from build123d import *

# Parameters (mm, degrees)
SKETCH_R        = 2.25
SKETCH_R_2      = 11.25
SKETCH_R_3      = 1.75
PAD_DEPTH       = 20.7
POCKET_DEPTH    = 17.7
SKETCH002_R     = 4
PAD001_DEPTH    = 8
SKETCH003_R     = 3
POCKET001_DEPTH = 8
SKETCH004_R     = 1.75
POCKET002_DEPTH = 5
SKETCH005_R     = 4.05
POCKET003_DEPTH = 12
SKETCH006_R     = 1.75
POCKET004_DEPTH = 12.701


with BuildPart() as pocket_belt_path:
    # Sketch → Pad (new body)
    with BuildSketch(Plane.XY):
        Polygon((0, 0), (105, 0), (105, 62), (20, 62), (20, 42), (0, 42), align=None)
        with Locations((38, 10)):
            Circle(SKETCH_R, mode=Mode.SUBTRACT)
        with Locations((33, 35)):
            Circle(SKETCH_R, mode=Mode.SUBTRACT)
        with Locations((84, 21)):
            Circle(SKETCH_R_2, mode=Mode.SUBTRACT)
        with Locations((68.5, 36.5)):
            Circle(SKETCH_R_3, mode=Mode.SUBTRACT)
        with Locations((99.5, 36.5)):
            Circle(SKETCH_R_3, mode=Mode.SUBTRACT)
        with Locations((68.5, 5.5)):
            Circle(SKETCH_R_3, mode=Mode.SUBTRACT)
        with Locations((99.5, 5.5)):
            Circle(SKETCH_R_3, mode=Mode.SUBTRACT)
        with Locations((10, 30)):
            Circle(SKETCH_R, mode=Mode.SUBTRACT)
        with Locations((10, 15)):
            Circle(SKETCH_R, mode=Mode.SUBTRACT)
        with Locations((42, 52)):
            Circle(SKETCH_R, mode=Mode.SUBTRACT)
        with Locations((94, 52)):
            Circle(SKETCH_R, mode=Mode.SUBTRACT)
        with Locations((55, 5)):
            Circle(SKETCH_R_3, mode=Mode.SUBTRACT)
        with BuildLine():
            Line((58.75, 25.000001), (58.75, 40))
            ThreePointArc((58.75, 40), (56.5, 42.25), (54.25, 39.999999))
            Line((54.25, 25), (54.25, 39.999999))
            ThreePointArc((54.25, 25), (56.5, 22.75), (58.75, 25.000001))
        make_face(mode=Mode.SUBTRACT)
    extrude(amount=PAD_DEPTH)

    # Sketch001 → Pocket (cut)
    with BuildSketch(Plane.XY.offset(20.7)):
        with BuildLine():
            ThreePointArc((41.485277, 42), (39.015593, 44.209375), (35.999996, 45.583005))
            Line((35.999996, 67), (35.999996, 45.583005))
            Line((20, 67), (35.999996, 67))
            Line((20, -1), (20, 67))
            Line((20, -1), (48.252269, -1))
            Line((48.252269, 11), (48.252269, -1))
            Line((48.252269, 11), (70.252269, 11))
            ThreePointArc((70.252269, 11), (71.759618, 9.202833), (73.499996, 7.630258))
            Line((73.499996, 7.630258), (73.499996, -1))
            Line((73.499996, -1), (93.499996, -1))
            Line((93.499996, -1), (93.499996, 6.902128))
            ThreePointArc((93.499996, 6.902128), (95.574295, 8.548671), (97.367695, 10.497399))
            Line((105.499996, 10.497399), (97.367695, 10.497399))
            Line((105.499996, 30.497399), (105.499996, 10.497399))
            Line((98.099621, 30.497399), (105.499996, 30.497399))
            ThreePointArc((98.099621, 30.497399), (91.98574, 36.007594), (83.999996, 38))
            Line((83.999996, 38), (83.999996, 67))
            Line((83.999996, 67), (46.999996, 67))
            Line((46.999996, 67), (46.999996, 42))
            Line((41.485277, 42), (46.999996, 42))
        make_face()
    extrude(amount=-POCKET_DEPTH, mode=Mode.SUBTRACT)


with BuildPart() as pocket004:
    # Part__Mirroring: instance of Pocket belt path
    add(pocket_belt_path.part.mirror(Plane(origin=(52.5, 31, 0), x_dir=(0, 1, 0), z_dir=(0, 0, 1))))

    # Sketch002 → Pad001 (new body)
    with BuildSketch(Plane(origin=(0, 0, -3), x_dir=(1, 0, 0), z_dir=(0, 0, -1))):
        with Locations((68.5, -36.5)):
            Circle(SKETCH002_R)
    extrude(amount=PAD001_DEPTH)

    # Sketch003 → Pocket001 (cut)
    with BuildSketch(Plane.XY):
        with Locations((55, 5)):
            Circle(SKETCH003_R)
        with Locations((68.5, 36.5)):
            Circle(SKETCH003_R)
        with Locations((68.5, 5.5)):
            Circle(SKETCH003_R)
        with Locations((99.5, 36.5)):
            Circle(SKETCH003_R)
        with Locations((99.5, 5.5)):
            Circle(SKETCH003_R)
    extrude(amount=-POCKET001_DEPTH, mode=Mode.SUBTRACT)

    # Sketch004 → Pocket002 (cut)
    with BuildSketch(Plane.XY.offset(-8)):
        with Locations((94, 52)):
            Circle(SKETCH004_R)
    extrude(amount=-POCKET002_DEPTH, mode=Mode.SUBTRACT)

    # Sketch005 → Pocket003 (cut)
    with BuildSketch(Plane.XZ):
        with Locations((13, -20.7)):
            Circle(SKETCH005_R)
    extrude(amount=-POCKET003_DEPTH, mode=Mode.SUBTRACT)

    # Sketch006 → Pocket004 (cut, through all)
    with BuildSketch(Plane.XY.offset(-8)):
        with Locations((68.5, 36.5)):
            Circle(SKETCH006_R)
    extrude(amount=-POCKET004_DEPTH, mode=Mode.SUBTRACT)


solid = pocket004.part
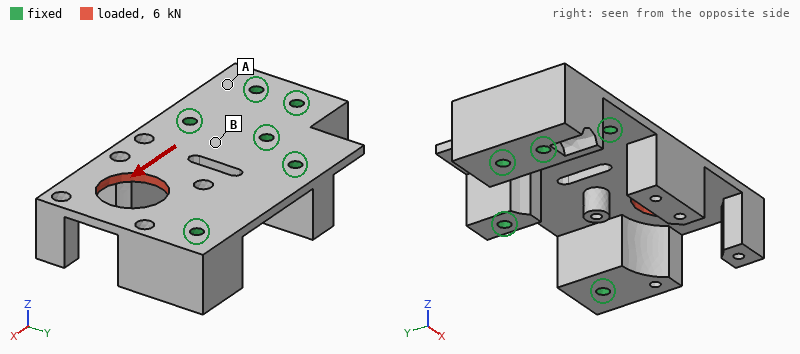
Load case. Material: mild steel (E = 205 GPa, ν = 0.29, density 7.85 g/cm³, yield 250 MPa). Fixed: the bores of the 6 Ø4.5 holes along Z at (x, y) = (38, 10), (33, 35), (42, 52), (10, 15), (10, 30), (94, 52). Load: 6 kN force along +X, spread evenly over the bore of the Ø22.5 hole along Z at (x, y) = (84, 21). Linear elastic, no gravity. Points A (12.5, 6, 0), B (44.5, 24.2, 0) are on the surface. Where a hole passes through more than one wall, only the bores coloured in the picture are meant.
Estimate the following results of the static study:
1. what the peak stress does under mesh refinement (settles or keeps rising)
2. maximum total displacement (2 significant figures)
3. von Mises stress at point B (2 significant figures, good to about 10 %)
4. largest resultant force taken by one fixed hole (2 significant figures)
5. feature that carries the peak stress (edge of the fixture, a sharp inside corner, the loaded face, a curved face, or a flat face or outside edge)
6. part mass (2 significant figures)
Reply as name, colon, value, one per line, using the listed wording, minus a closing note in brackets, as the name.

what the peak stress does under mesh refinement: keeps rising
maximum total displacement: 17 µm
von Mises stress at point B: 18 MPa
largest resultant force taken by one fixed hole: 2.4 kN
feature that carries the peak stress: a sharp inside corner
part mass: 390 g
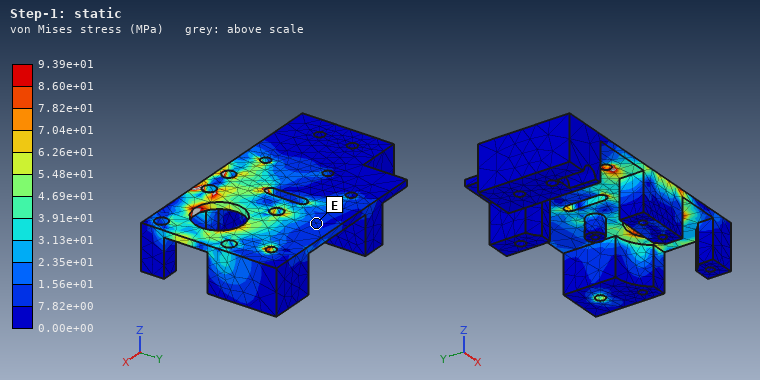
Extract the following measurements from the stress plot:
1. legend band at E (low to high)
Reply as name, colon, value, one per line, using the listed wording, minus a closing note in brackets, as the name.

legend band at E: 7.82e+00 to 1.56e+01 MPa
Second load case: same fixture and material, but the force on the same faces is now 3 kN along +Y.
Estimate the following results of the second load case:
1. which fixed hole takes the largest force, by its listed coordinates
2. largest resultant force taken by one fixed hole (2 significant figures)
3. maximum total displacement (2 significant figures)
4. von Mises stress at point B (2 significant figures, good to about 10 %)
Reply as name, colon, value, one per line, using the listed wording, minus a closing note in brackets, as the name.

which fixed hole takes the largest force, by its listed coordinates: (94, 52)
largest resultant force taken by one fixed hole: 2.2 kN
maximum total displacement: 11 µm
von Mises stress at point B: 13 MPa
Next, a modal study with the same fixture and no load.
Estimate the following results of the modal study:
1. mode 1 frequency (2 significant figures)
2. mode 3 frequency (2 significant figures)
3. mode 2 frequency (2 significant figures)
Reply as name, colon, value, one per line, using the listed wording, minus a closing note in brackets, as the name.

mode 1 frequency: 1200 Hz
mode 3 frequency: 3700 Hz
mode 2 frequency: 2200 Hz
